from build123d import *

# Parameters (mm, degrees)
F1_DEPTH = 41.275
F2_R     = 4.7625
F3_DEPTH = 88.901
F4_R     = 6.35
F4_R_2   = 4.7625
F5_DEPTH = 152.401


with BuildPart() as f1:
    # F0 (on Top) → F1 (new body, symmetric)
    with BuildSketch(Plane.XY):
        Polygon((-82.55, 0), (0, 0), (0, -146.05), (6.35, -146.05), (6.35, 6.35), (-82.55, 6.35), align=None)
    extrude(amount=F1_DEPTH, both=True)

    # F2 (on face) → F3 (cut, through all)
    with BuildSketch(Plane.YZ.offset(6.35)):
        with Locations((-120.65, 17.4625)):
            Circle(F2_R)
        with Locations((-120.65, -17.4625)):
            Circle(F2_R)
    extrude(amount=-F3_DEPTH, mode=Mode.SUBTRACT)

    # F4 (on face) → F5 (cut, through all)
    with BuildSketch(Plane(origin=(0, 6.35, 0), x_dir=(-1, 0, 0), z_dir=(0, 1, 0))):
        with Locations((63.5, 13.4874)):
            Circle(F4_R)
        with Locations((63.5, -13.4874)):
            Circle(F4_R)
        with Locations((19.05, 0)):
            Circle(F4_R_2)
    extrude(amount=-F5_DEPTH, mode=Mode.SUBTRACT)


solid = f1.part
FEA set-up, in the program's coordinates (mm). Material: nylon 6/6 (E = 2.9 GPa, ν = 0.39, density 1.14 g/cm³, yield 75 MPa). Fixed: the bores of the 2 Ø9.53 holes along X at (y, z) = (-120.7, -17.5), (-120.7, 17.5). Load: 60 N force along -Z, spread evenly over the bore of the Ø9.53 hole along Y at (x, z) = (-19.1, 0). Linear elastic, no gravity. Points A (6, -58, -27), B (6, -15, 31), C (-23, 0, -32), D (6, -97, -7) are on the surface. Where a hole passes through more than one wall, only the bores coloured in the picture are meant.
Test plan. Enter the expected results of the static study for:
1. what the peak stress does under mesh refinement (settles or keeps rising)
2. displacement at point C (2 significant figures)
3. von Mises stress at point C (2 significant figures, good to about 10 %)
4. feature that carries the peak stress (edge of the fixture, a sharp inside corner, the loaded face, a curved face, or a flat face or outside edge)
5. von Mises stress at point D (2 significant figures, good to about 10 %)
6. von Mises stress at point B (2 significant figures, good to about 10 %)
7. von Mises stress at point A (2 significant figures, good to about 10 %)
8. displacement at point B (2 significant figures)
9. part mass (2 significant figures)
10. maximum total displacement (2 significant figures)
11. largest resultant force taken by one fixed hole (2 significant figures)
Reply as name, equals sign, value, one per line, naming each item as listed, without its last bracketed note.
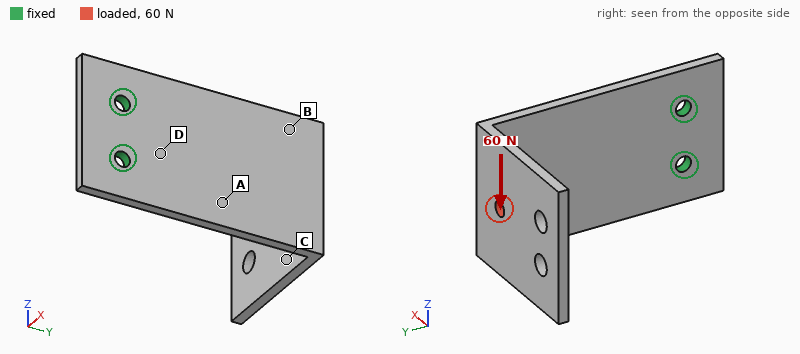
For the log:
what the peak stress does under mesh refinement = keeps rising
displacement at point C = 0.79 mm
von Mises stress at point C = 0.55 MPa
feature that carries the peak stress = edge of the fixture
von Mises stress at point D = 1.2 MPa
von Mises stress at point B = 1.6 MPa
von Mises stress at point A = 1.9 MPa
displacement at point B = 0.49 mm
part mass = 140 g
maximum total displacement = 1.8 mm
largest resultant force taken by one fixed hole = 180 N
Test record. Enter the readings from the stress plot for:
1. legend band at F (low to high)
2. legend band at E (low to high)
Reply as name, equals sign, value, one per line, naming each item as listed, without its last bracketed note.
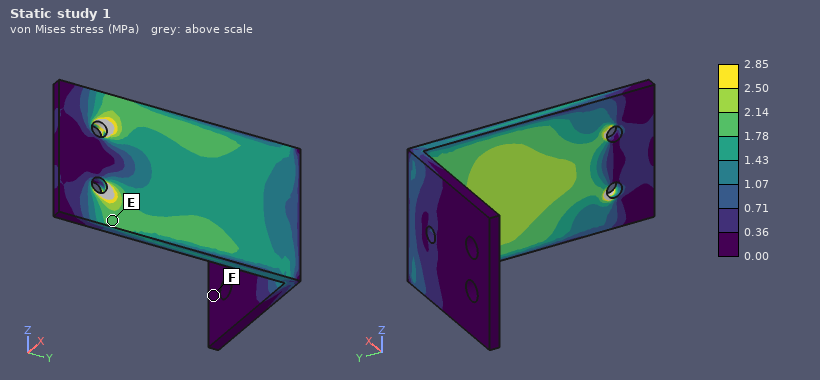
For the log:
legend band at F = 0.00 to 0.36 MPa
legend band at E = 1.78 to 2.14 MPa
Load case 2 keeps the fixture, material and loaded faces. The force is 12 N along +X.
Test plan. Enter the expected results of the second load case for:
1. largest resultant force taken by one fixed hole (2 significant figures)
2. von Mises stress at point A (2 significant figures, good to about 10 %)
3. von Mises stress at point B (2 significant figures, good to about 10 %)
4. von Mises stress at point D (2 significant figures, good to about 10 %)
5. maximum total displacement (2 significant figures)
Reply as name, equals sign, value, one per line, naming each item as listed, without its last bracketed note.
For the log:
largest resultant force taken by one fixed hole = 6.0 N
von Mises stress at point A = 1.3 MPa
von Mises stress at point B = 0.46 MPa
von Mises stress at point D = 2.0 MPa
maximum total displacement = 2.0 mm
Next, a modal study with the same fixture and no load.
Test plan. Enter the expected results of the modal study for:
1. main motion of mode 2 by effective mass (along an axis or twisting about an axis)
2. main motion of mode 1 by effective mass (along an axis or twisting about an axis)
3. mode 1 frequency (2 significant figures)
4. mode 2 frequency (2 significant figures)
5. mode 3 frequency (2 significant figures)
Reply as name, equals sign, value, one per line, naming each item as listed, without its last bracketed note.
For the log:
main motion of mode 2 by effective mass = along Z
main motion of mode 1 by effective mass = along X
mode 1 frequency = 51 Hz
mode 2 frequency = 110 Hz
mode 3 frequency = 170 Hz
